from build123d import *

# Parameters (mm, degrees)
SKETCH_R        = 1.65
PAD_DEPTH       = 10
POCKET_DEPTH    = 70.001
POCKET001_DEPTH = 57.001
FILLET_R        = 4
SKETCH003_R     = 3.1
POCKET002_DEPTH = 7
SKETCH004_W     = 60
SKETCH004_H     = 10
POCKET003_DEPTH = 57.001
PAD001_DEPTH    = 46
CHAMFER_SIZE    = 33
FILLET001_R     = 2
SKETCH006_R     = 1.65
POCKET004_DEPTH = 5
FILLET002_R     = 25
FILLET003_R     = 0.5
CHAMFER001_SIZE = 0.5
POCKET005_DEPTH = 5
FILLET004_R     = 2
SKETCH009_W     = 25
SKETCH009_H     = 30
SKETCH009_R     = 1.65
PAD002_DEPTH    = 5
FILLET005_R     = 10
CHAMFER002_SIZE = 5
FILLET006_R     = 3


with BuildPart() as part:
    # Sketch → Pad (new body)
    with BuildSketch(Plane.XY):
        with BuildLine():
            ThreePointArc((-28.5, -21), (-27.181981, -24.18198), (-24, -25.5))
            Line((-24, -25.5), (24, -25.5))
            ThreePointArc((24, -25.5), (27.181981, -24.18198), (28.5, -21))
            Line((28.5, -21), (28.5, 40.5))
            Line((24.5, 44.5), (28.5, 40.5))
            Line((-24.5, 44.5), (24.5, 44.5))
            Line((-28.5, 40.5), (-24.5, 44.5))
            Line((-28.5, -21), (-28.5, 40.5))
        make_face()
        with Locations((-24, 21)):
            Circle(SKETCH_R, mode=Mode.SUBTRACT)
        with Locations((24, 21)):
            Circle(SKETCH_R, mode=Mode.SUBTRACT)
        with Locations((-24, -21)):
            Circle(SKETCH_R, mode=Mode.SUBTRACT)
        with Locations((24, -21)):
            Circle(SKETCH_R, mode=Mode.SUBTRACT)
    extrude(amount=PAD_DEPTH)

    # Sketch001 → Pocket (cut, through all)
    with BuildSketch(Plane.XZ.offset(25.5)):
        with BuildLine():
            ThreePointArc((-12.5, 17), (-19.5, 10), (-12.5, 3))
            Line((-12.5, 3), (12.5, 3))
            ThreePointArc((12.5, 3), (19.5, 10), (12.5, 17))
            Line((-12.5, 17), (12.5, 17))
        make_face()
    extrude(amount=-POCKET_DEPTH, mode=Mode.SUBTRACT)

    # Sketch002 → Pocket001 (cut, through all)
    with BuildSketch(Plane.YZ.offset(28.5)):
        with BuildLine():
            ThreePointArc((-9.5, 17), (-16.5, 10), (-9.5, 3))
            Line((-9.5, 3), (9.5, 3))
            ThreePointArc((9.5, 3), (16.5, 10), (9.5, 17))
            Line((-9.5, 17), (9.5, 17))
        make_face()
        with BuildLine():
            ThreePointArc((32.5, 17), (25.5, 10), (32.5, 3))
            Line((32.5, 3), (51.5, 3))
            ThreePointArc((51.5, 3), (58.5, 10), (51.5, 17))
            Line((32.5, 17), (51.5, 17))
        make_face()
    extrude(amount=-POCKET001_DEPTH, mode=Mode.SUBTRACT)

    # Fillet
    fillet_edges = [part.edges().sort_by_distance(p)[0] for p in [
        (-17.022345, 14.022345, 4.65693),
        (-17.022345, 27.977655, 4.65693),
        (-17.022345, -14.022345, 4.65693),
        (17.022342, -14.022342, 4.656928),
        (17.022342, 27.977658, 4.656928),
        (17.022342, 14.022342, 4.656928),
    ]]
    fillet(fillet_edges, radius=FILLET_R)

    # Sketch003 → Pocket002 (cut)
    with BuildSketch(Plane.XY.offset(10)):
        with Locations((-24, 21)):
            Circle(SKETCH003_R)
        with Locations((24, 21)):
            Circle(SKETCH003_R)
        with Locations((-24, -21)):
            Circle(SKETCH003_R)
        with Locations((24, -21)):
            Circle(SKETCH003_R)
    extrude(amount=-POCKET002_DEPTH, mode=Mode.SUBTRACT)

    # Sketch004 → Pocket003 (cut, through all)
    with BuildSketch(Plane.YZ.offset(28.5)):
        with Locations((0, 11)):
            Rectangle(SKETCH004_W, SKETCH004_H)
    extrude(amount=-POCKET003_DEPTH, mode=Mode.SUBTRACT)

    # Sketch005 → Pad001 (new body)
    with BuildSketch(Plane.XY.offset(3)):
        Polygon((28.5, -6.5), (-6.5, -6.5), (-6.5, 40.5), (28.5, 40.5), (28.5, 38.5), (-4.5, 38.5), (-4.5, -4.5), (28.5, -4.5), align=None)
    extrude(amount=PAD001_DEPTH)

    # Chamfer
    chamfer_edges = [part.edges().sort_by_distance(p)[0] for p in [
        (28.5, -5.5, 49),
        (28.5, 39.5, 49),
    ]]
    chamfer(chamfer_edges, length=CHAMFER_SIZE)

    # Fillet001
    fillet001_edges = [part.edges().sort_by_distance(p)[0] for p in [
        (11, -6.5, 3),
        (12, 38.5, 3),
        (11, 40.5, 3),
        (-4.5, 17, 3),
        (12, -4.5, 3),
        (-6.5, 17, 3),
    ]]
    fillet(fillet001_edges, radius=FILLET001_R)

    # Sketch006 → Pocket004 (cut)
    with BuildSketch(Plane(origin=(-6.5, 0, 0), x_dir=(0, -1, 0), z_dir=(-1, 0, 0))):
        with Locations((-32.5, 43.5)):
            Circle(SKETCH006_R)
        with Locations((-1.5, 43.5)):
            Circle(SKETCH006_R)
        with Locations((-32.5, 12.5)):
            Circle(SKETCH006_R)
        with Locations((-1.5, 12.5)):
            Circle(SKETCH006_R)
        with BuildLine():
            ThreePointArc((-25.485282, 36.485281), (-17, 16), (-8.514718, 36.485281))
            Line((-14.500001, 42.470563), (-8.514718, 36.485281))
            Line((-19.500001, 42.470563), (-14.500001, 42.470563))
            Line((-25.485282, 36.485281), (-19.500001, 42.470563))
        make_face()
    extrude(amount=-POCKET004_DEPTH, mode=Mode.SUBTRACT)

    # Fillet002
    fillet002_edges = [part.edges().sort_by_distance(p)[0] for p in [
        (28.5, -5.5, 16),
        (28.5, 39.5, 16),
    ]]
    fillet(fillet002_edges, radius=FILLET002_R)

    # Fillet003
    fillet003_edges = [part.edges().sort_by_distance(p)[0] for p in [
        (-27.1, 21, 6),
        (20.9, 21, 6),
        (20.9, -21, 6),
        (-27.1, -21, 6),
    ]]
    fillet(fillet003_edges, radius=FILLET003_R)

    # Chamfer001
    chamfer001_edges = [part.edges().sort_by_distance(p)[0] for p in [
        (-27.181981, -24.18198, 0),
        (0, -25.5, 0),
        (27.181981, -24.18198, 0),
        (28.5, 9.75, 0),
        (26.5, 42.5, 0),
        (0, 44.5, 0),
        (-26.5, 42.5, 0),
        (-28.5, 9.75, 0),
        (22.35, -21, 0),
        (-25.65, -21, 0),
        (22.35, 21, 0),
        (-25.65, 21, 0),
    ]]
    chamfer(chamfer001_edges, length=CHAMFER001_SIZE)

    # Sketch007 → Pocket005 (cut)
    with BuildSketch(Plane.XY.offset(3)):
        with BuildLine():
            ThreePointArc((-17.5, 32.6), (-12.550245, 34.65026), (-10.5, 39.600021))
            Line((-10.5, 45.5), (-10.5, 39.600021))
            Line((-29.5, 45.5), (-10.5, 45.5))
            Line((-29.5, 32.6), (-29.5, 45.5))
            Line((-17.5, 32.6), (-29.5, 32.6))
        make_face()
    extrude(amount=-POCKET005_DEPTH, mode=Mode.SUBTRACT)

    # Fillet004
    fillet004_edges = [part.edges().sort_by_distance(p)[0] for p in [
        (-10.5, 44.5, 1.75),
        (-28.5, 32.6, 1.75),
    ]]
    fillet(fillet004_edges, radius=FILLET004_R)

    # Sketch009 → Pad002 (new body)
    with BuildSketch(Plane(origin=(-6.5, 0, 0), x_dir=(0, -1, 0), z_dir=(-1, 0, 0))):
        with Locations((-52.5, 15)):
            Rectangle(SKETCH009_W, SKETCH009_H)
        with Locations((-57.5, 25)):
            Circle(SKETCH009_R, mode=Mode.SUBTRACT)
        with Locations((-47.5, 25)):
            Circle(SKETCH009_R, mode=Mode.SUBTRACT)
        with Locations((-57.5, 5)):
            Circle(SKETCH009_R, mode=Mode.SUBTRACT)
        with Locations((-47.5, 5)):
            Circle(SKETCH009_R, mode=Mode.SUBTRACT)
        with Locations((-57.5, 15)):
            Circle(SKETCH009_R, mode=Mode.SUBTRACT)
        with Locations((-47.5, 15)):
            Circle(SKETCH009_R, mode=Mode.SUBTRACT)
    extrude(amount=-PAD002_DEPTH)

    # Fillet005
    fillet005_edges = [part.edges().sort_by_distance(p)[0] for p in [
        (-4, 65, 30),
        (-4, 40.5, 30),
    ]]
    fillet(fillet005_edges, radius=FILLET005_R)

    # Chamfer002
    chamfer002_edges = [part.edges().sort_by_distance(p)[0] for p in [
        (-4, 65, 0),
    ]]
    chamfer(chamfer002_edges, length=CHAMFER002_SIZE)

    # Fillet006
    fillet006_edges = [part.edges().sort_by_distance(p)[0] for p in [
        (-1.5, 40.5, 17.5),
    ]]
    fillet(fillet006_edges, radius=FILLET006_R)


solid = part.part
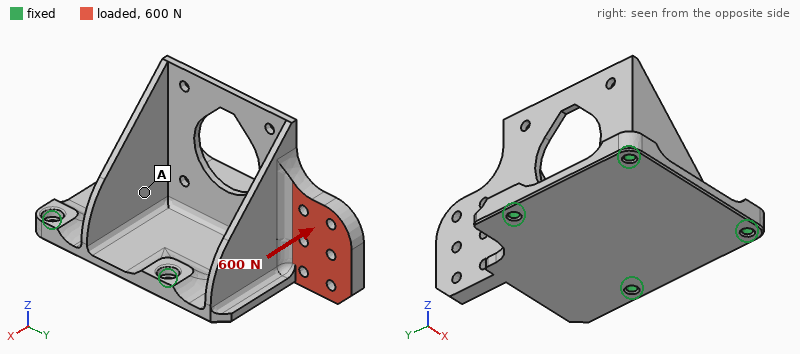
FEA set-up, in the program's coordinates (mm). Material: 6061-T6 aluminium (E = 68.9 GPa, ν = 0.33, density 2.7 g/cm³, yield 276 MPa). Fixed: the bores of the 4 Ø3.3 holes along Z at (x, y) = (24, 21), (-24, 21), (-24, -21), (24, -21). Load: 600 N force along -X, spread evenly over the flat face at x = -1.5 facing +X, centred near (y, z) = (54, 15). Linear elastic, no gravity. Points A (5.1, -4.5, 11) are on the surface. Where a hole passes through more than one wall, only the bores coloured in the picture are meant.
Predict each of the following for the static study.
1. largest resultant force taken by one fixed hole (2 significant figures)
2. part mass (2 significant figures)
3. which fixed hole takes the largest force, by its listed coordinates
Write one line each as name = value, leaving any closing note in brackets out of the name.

largest resultant force taken by one fixed hole = 610 N
part mass = 63 g
which fixed hole takes the largest force, by its listed coordinates = (24, 21)
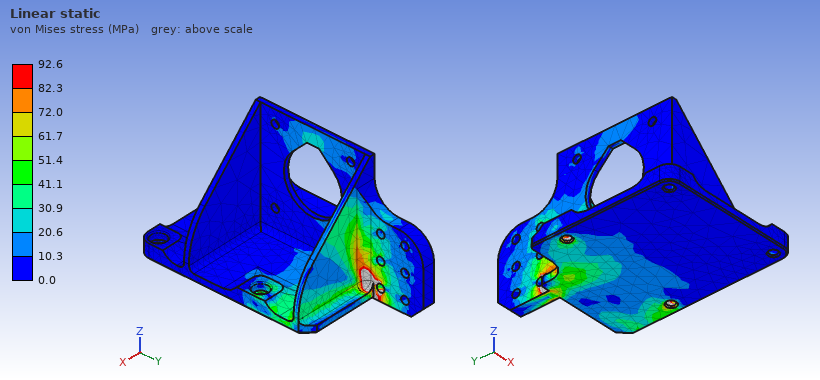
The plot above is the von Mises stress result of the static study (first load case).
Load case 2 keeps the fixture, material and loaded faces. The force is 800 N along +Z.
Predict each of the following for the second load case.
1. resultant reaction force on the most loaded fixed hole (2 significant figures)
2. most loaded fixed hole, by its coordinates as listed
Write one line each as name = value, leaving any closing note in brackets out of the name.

resultant reaction force on the most loaded fixed hole = 760 N
most loaded fixed hole, by its coordinates as listed = (-24, 21)
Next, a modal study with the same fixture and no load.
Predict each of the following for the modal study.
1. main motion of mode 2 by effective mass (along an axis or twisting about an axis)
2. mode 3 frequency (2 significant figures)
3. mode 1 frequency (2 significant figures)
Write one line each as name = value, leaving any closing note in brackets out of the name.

main motion of mode 2 by effective mass = along X
mode 3 frequency = 3500 Hz
mode 1 frequency = 1700 Hz
